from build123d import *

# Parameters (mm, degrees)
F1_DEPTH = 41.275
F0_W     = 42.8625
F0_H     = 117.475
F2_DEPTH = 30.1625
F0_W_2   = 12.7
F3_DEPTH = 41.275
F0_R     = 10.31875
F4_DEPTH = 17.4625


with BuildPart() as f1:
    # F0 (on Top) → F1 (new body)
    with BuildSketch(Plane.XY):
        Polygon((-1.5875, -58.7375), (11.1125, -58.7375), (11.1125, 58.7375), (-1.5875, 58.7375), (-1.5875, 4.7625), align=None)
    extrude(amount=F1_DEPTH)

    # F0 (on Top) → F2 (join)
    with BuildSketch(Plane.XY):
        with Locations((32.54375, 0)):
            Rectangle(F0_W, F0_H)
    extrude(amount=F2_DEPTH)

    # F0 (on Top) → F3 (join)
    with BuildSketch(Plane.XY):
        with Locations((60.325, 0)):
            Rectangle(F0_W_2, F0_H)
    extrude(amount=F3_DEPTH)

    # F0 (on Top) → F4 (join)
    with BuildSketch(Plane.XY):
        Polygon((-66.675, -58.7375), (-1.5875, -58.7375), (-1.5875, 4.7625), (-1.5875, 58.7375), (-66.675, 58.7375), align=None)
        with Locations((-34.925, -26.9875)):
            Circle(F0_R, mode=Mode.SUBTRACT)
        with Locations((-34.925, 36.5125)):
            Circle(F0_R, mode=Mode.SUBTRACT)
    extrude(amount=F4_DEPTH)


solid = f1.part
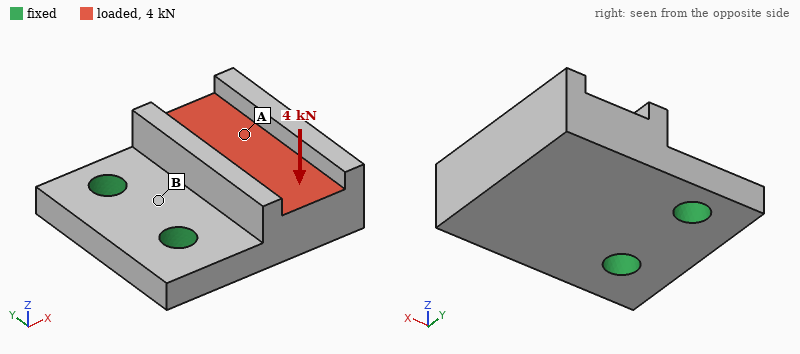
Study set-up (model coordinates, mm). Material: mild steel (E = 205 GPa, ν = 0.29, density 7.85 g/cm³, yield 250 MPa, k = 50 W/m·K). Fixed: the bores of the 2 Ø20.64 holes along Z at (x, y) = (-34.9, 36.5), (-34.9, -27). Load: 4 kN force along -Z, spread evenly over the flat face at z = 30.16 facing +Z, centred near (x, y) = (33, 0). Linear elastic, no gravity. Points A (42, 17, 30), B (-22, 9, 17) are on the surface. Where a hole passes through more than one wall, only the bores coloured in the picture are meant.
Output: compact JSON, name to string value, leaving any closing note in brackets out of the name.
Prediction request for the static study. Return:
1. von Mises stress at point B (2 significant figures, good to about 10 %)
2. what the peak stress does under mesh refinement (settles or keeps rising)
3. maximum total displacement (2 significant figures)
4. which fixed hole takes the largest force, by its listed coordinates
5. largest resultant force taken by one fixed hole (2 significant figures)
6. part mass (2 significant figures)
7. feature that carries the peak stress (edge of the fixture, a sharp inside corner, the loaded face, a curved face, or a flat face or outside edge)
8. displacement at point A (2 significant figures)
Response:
{"von Mises stress at point B": "22 MPa", "what the peak stress does under mesh refinement": "keeps rising", "maximum total displacement": "55 µm", "which fixed hole takes the largest force, by its listed coordinates": "(-34.9, -27)", "largest resultant force taken by one fixed hole": "2.2 kN", "part mass": "3.1 kg", "feature that carries the peak stress": "edge of the fixture", "displacement at point A": "38 µm"}
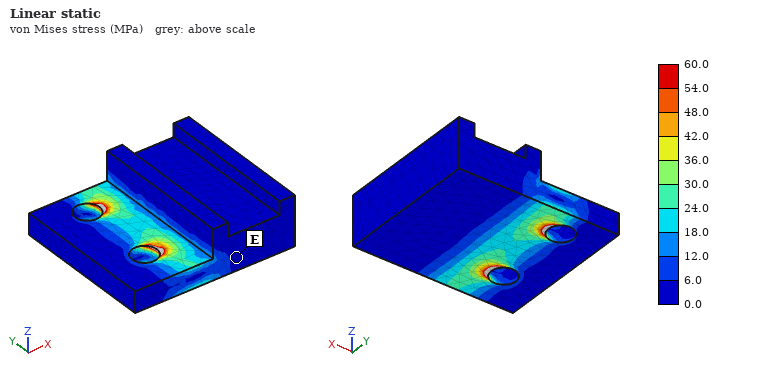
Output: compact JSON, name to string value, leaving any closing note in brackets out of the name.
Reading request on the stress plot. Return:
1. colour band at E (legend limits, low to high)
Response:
{"colour band at E": "0.0 to 6.0 MPa"}
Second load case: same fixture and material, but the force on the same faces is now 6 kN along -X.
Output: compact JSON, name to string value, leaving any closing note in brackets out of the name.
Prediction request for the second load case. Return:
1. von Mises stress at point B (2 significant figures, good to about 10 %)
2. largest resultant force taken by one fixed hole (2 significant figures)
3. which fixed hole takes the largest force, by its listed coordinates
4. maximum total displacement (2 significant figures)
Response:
{"von Mises stress at point B": "16 MPa", "largest resultant force taken by one fixed hole": "3.4 kN", "which fixed hole takes the largest force, by its listed coordinates": "(-34.9, -27)", "maximum total displacement": "38 µm"}
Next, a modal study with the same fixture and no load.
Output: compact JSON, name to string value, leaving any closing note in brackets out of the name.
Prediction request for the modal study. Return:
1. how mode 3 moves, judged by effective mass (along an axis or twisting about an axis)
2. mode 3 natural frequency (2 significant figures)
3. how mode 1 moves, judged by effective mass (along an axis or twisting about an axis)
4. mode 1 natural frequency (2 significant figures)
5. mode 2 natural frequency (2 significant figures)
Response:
{"how mode 3 moves, judged by effective mass": "along Y", "mode 3 natural frequency": "4100 Hz", "how mode 1 moves, judged by effective mass": "along Z", "mode 1 natural frequency": "1100 Hz", "mode 2 natural frequency": "3000 Hz"}
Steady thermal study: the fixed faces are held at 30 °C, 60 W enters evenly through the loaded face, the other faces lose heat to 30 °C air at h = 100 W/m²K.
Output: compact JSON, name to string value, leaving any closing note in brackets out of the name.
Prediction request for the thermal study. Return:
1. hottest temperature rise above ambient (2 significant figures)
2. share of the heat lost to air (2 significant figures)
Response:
{"hottest temperature rise above ambient": "17 K", "share of the heat lost to air": "58 %"}
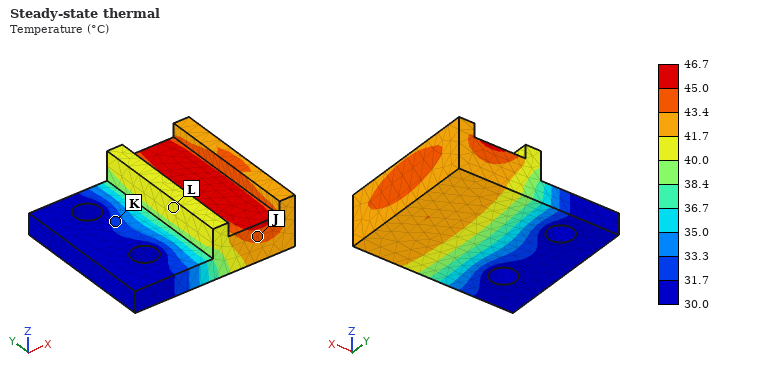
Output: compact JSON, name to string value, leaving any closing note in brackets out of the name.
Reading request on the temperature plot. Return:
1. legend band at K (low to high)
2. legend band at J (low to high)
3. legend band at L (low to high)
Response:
{"legend band at K": "31.7 to 33.3 °C", "legend band at J": "43.4 to 45.0 °C", "legend band at L": "40.0 to 41.7 °C"}
